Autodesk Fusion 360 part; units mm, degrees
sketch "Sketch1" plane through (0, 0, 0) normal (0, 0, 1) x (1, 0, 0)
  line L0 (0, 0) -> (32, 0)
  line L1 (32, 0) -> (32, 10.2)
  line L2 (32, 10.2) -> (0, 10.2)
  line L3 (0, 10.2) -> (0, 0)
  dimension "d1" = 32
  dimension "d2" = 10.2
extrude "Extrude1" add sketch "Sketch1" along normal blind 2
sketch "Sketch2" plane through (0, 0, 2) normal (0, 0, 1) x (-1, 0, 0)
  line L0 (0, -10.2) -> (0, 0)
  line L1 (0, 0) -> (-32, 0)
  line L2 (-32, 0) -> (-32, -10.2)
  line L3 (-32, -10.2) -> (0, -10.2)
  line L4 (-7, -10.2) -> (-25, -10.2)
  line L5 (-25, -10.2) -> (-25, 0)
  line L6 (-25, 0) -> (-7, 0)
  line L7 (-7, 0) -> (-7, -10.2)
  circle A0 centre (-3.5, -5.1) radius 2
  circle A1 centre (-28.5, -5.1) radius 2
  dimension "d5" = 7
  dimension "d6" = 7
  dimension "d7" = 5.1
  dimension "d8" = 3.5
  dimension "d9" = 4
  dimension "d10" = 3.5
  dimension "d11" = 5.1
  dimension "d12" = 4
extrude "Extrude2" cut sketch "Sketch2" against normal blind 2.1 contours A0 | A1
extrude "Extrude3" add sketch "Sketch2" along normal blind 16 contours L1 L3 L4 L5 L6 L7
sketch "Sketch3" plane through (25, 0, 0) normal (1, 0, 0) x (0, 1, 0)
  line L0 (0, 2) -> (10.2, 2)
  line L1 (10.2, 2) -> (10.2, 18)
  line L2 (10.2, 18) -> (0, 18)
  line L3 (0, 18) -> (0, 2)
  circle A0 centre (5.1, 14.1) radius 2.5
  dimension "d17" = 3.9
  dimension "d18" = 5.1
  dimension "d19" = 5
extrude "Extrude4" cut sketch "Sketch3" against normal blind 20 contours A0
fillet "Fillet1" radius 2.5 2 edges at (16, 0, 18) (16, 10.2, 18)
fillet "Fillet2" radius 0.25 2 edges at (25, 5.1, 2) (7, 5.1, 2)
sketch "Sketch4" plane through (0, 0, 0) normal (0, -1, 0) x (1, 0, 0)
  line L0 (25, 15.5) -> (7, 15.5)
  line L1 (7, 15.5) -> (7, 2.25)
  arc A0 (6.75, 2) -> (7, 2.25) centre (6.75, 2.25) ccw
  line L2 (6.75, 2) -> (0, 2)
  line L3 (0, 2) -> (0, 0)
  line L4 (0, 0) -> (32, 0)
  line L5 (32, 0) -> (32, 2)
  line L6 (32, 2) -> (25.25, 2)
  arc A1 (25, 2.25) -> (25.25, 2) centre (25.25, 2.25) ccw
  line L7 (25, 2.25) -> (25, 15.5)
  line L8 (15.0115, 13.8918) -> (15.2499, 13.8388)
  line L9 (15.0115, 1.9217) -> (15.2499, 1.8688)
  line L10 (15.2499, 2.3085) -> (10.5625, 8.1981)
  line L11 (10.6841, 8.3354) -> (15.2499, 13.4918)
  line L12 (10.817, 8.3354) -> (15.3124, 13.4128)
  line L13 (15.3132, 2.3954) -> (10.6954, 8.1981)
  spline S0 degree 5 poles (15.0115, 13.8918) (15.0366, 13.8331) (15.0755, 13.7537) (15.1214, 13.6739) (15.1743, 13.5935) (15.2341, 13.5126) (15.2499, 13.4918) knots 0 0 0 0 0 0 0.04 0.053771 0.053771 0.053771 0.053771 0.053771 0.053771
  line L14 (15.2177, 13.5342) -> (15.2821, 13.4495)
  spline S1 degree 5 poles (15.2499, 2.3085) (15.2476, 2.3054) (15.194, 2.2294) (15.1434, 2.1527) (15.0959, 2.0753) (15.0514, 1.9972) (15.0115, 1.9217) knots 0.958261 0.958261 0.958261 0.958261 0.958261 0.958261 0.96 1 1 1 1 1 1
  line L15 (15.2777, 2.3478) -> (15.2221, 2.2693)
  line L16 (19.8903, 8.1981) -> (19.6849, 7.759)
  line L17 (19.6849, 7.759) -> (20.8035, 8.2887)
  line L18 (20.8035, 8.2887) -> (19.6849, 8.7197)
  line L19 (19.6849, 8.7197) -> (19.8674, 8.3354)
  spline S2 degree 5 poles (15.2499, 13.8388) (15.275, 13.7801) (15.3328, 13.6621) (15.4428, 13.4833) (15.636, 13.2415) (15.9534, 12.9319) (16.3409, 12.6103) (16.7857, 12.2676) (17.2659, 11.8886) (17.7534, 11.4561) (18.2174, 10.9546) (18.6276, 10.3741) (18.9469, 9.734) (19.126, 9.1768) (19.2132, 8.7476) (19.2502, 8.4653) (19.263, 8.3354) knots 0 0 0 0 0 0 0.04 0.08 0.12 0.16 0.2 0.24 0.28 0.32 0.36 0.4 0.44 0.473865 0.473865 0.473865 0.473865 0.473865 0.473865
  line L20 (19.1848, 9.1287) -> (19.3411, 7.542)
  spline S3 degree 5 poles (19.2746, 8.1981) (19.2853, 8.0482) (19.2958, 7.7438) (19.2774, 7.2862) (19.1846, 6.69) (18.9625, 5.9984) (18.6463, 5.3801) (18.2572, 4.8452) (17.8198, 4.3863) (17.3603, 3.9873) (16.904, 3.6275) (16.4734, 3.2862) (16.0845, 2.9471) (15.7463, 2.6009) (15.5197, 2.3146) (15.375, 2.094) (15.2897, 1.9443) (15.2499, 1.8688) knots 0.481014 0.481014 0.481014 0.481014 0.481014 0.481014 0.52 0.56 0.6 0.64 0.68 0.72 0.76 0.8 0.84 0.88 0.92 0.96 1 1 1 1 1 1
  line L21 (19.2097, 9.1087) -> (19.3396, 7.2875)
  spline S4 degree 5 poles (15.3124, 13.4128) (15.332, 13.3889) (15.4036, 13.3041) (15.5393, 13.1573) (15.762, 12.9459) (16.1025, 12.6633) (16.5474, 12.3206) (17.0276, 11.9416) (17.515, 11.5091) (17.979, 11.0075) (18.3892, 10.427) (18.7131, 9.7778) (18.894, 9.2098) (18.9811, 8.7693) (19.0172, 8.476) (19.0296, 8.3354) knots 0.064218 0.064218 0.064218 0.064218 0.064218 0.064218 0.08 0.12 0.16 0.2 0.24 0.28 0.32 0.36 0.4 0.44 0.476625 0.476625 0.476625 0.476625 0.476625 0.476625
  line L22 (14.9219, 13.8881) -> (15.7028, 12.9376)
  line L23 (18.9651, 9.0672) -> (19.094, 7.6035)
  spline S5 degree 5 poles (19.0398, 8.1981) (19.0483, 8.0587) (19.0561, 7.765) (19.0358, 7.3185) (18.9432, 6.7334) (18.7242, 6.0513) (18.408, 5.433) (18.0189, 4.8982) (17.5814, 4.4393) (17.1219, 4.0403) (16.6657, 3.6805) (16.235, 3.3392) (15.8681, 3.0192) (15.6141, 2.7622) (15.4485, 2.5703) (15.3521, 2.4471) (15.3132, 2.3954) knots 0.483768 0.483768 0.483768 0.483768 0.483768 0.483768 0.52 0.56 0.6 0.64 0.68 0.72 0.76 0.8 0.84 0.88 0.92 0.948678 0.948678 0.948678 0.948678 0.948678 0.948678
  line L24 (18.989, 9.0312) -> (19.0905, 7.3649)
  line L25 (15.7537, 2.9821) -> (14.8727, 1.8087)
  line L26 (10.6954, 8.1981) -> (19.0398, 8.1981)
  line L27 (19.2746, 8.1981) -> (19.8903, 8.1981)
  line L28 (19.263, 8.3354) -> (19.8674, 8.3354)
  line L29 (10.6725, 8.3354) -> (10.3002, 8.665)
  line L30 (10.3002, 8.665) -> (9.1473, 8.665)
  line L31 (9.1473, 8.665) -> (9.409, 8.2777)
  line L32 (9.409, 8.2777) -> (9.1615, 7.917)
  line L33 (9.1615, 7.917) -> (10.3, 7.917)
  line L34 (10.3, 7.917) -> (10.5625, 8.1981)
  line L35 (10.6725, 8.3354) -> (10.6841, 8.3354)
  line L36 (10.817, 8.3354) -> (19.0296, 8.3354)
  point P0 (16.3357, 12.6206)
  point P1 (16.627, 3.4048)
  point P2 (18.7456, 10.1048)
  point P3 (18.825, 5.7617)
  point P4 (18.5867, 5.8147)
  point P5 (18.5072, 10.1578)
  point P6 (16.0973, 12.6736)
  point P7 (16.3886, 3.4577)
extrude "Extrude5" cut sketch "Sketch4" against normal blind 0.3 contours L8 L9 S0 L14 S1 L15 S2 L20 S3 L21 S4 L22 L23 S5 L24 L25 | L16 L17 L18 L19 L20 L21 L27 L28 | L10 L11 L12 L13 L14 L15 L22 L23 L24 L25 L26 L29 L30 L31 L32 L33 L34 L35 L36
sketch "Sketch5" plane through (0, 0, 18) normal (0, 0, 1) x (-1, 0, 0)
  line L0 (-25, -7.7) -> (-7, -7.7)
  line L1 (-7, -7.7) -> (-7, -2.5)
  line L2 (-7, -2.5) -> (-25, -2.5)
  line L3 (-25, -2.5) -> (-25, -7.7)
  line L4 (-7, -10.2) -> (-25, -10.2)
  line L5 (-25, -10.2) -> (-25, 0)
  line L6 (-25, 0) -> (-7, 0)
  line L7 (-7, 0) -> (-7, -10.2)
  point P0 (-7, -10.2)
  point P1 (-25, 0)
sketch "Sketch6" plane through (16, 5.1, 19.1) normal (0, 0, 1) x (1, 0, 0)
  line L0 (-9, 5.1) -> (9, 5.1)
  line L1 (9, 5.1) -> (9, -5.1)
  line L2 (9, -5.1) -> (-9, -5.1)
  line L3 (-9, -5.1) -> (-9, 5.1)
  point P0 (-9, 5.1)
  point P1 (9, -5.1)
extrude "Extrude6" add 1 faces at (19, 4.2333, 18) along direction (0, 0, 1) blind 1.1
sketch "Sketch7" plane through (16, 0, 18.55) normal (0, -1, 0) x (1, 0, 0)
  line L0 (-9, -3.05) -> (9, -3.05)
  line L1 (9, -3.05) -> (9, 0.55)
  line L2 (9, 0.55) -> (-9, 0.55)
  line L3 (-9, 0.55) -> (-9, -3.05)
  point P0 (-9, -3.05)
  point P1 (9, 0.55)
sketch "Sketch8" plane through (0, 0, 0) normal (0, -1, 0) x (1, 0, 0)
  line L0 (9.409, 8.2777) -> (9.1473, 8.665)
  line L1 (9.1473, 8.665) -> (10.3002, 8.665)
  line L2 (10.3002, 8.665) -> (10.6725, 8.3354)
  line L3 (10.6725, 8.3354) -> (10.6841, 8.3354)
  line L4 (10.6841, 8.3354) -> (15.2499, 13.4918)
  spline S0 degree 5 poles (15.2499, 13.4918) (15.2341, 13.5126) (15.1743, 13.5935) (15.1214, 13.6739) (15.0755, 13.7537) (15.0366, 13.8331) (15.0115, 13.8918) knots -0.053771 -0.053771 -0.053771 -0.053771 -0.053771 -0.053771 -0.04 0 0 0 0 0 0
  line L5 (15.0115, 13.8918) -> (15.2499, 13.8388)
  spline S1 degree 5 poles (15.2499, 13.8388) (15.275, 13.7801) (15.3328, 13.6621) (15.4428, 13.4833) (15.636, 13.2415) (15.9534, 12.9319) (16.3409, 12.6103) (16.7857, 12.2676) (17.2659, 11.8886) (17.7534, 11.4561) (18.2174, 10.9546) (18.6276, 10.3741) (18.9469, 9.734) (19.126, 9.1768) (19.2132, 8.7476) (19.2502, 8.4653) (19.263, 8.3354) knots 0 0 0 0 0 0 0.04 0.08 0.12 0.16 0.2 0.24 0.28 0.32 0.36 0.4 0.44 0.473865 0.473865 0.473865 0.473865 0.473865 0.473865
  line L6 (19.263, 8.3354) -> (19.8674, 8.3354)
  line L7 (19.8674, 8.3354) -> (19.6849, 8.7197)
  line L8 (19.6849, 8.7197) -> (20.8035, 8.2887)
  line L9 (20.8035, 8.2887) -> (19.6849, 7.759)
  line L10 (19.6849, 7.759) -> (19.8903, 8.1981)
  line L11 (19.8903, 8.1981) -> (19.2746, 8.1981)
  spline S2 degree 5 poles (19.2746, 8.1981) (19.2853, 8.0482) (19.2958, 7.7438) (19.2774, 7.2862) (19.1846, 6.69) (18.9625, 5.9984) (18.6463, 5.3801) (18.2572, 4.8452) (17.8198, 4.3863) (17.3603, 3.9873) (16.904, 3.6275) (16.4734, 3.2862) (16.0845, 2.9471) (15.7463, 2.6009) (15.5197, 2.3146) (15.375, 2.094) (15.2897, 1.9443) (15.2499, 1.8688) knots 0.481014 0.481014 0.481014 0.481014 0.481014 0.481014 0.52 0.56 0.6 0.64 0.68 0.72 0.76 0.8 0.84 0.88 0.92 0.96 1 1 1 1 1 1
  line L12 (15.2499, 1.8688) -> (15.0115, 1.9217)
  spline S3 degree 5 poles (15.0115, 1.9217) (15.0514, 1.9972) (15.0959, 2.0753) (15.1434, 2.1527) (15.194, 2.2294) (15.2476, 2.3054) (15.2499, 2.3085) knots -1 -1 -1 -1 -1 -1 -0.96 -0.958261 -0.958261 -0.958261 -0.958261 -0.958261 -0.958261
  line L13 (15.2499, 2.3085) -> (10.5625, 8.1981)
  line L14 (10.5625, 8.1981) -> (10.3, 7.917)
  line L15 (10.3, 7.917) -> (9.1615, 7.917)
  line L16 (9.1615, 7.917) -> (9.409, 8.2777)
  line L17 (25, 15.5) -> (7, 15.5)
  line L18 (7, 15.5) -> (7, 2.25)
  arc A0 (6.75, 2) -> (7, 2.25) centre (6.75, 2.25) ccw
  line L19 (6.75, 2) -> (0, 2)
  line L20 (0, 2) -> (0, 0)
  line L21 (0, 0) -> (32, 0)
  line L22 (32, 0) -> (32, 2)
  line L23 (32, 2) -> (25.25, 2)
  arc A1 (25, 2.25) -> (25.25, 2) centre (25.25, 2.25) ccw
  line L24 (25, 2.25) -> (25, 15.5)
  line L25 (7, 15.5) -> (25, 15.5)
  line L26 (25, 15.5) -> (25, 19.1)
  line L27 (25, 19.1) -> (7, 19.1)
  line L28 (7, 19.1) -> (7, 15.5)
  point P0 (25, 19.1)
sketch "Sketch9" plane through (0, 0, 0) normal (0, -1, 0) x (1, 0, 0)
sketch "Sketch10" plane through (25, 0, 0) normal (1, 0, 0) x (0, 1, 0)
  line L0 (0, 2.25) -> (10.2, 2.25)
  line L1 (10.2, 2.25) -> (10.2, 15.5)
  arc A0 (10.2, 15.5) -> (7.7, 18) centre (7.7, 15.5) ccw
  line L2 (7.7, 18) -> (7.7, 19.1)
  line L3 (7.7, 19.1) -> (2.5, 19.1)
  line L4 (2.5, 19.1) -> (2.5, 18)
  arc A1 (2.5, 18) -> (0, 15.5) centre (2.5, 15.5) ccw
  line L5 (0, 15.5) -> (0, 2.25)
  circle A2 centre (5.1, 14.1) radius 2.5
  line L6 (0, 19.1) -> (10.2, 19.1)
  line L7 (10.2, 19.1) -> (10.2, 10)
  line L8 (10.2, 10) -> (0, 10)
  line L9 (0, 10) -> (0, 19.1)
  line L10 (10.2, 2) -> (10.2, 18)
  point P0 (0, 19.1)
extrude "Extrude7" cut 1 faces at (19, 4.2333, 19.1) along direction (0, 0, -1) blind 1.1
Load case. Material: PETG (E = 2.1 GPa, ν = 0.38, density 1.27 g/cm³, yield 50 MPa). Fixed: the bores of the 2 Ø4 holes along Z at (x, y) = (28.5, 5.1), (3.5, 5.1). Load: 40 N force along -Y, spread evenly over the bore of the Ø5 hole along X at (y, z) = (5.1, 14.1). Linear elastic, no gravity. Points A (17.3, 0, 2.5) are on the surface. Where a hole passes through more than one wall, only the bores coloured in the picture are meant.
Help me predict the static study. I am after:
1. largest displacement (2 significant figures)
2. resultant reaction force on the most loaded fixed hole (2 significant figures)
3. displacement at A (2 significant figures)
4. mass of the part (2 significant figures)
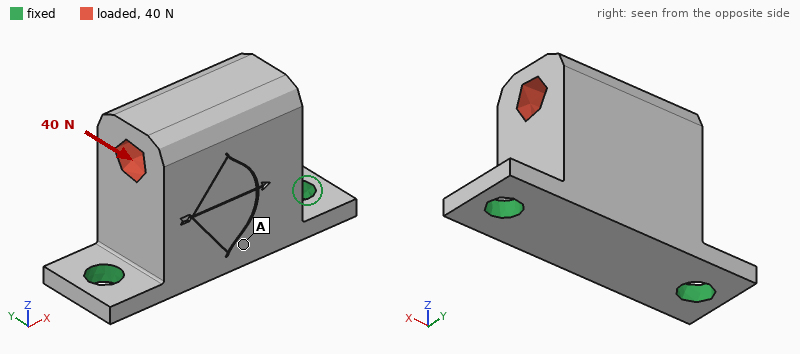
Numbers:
0.40 mm
20 N
0.12 mm
4.0 g
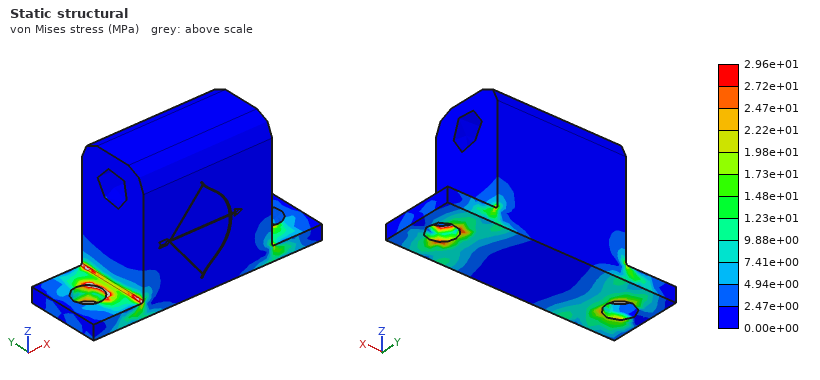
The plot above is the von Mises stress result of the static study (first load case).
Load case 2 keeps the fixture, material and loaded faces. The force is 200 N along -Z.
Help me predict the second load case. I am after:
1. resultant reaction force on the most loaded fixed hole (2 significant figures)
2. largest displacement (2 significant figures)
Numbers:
110 N
65 µm
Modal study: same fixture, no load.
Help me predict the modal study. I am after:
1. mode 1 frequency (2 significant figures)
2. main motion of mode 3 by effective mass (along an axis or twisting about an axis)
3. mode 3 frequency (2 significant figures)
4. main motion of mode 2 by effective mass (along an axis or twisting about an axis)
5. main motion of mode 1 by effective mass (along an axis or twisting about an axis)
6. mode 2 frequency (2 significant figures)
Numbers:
1300 Hz
along Z
5000 Hz
along X
along Y
4700 Hz
